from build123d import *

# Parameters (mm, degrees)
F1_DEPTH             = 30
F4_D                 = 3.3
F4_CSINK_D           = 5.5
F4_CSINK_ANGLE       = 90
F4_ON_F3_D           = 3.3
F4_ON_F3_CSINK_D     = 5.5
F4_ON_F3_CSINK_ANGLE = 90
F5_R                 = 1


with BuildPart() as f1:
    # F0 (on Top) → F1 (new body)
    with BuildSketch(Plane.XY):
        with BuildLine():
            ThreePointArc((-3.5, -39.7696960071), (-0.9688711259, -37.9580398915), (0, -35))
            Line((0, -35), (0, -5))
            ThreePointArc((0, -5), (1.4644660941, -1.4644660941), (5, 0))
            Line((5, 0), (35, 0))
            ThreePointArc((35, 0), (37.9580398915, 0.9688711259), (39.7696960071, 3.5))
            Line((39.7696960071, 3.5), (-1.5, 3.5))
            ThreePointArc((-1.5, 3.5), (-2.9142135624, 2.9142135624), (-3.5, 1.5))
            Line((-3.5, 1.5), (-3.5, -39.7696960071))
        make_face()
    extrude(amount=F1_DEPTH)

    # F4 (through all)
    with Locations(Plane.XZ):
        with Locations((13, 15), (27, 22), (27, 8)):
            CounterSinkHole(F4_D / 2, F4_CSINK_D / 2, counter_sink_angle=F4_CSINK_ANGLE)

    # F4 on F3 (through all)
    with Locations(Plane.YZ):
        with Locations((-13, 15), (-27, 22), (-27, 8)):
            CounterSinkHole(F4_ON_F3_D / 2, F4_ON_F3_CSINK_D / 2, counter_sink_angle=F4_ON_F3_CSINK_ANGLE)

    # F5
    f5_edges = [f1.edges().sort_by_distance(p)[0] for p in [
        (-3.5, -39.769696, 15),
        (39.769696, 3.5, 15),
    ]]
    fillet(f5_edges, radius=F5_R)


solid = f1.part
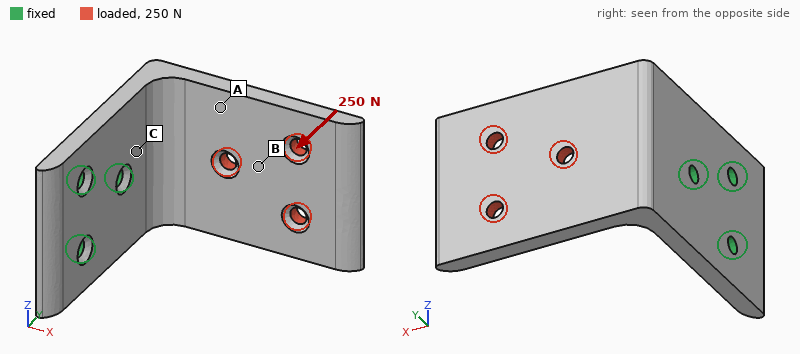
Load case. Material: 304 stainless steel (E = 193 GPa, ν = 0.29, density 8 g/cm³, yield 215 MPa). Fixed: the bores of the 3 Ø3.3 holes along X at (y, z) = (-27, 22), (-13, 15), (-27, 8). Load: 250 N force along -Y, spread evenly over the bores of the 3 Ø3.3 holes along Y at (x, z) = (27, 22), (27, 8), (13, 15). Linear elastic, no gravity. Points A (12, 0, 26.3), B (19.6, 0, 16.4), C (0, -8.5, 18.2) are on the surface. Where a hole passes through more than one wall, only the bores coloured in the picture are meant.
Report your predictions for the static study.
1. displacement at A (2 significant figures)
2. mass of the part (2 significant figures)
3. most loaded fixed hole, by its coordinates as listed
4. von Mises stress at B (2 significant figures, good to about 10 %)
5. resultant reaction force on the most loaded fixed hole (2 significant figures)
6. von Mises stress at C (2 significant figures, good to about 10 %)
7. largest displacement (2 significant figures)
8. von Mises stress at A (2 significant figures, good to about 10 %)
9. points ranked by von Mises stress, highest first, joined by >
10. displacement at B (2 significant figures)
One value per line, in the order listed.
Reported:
0.070 mm
67 g
(-13, 15)
19 MPa
300 N
100 MPa
0.25 mm
45 MPa
C > A > B
0.11 mm
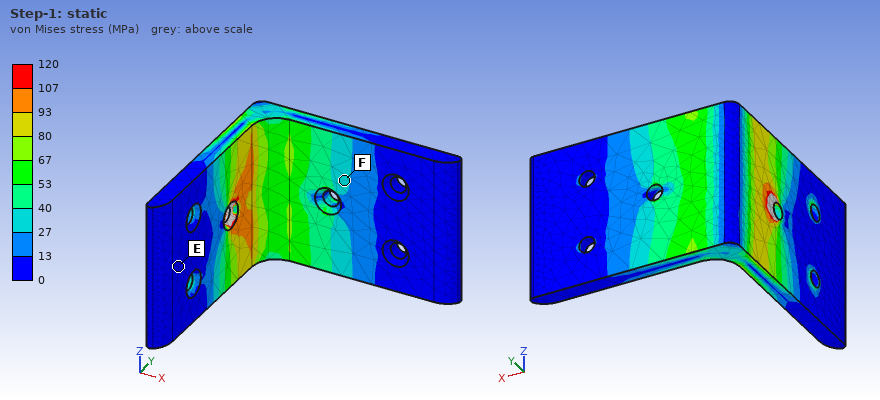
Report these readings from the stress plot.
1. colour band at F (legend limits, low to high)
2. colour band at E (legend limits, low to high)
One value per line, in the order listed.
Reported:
27 to 40 MPa
0 to 13 MPa
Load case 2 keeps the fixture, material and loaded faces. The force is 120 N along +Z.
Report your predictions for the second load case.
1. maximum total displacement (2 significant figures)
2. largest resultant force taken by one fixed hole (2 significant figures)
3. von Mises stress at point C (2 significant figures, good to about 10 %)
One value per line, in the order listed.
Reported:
52 µm
130 N
31 MPa
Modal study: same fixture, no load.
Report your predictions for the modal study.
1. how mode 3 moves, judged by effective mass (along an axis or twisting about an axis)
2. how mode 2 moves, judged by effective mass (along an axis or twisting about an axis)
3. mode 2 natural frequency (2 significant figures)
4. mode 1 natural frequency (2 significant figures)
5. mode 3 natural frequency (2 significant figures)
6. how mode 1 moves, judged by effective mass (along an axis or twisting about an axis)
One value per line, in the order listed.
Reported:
along X
along Z
1700 Hz
1200 Hz
4300 Hz
along Y
